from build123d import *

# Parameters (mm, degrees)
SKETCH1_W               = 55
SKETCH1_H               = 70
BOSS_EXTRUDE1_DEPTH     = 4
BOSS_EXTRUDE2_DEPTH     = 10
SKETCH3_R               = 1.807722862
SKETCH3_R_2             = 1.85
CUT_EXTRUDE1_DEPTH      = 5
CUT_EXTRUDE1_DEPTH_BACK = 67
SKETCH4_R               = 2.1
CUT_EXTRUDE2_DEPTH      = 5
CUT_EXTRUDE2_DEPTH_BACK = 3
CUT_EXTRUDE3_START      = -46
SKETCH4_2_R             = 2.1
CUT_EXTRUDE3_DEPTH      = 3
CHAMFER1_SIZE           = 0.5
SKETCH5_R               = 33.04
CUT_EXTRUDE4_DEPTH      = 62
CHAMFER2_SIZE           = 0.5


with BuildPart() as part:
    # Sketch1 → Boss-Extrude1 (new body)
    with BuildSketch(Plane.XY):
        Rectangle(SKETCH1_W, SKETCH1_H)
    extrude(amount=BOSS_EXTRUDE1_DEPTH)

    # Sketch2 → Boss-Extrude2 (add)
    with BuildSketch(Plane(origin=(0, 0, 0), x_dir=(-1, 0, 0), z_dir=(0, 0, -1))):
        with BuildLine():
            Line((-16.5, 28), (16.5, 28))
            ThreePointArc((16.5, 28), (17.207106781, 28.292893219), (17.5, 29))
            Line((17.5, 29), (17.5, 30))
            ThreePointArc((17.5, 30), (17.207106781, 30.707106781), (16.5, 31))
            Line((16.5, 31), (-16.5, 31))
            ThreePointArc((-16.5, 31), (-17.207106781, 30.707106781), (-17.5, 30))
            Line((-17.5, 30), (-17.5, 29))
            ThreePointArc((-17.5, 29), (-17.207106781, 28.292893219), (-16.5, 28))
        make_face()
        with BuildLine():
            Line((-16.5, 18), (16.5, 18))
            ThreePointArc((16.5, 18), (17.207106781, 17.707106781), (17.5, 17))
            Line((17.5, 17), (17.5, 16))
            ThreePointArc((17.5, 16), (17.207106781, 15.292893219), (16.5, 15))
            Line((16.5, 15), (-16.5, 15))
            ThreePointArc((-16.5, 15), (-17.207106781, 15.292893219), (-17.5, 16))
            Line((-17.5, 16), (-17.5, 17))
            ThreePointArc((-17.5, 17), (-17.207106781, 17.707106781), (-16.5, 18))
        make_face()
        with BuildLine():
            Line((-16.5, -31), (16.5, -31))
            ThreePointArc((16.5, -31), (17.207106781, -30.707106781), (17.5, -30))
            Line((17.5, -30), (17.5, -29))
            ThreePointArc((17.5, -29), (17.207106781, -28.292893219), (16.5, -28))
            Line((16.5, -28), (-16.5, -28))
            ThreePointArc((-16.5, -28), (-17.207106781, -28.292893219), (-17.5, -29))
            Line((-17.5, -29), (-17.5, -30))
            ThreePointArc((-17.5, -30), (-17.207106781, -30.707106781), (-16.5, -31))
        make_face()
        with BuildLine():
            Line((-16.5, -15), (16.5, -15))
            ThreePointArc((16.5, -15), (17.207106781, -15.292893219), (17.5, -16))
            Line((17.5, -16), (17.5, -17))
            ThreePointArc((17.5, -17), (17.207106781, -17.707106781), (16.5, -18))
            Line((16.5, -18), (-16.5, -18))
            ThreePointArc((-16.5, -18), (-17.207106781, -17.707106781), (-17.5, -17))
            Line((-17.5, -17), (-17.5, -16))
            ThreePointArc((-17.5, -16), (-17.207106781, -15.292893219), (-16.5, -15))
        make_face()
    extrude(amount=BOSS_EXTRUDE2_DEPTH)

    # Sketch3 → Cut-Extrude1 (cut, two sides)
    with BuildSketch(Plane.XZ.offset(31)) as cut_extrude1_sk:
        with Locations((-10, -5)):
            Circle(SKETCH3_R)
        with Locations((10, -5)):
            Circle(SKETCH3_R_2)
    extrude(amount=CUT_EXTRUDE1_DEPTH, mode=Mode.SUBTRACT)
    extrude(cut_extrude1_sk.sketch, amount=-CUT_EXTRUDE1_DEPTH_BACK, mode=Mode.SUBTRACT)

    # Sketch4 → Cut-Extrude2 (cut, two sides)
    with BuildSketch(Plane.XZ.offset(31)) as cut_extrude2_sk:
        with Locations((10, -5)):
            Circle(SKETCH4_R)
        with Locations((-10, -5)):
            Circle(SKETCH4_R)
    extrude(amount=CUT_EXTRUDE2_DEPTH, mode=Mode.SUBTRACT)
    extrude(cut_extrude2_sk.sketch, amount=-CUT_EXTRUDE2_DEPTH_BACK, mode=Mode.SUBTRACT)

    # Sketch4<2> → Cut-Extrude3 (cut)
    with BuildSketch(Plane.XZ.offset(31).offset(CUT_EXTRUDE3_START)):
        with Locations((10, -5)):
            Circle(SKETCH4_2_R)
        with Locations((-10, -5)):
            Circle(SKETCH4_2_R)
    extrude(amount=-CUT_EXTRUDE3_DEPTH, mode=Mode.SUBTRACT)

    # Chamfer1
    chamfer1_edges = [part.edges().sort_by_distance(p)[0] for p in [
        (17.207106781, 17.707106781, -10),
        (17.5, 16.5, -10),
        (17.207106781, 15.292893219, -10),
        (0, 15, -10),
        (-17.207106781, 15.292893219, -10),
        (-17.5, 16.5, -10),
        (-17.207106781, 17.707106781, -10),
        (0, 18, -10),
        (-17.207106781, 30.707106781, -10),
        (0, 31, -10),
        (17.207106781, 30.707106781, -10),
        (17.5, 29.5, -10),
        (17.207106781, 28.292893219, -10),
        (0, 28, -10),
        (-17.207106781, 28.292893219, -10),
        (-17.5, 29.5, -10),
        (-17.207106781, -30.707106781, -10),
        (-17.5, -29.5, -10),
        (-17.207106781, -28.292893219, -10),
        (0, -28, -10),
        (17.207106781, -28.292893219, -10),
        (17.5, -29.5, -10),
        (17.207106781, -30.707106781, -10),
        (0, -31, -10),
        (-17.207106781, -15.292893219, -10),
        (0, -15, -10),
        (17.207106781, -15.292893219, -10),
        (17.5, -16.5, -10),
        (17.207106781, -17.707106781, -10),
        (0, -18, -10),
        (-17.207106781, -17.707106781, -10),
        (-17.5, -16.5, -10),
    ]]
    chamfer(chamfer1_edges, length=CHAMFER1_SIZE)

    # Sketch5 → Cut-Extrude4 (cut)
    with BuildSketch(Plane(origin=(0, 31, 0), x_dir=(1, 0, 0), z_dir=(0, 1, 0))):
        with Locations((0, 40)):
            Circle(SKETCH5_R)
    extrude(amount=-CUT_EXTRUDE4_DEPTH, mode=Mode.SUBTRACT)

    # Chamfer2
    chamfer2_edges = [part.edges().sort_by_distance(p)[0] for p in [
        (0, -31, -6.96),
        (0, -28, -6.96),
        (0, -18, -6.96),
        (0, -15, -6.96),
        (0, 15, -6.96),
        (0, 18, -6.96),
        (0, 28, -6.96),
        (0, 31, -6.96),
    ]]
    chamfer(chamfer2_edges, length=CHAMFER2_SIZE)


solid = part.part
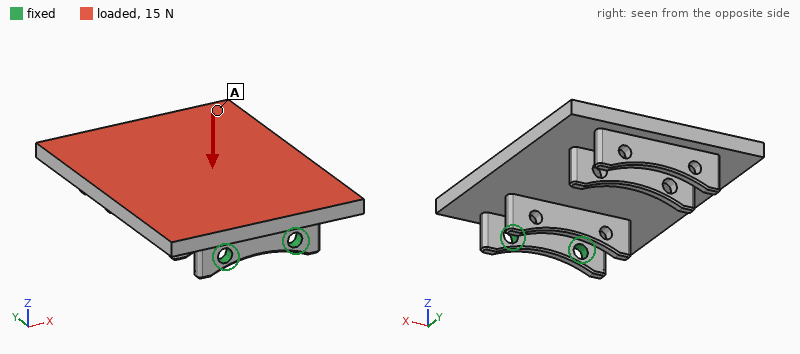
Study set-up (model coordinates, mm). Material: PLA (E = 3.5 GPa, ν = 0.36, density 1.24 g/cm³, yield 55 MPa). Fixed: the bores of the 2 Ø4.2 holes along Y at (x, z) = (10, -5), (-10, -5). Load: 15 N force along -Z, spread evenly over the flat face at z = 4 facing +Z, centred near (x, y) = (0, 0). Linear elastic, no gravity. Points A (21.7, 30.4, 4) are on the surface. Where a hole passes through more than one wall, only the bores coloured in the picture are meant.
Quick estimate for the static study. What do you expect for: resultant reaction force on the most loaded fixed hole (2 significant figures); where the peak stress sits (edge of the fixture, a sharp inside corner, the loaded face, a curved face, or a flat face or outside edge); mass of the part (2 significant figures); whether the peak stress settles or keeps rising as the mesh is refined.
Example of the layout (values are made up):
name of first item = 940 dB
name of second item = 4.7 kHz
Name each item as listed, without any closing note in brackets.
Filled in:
resultant reaction force on the most loaded fixed hole = 8.7 N
where the peak stress sits = edge of the fixture
mass of the part = 23 g
whether the peak stress settles or keeps rising as the mesh is refined = keeps rising
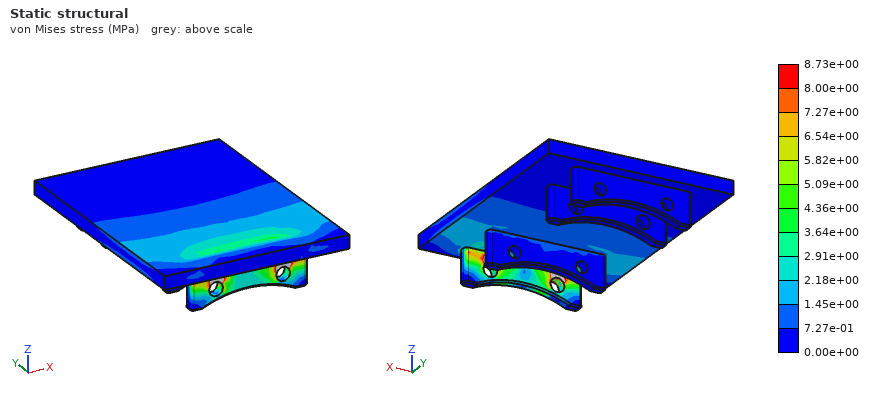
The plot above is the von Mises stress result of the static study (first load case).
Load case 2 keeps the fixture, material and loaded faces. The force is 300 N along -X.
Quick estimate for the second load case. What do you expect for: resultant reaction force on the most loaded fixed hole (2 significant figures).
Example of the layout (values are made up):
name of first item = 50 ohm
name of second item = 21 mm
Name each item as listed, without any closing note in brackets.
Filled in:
resultant reaction force on the most loaded fixed hole = 430 N
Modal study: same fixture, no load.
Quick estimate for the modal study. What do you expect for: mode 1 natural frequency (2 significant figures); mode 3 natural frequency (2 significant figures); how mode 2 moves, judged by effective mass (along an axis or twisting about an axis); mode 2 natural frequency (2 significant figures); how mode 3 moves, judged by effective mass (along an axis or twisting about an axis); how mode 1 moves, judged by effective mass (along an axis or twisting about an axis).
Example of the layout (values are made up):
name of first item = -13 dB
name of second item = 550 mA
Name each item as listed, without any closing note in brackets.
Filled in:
mode 1 natural frequency = 160 Hz
mode 3 natural frequency = 740 Hz
how mode 2 moves, judged by effective mass = along X
mode 2 natural frequency = 530 Hz
how mode 3 moves, judged by effective mass = along X
how mode 1 moves, judged by effective mass = along Z
